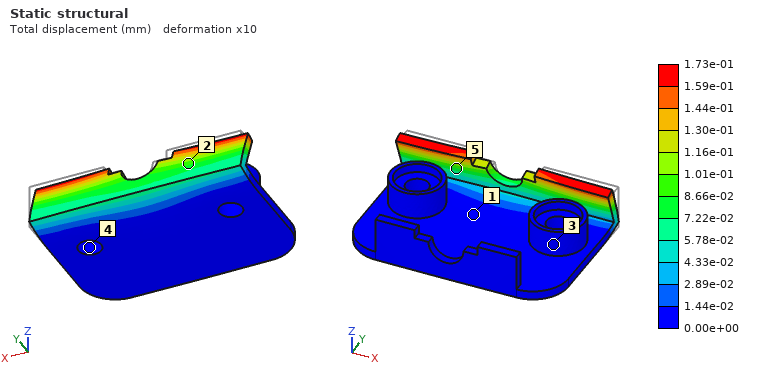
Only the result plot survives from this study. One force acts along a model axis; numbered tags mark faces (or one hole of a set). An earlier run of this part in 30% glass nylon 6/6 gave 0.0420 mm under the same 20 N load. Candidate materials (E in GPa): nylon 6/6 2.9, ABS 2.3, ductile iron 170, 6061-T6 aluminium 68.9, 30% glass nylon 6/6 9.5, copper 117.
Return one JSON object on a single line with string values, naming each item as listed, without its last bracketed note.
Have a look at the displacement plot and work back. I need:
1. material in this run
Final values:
{"material in this run": "ABS"}
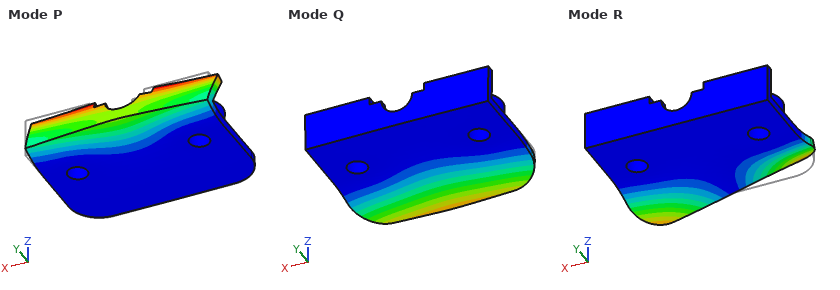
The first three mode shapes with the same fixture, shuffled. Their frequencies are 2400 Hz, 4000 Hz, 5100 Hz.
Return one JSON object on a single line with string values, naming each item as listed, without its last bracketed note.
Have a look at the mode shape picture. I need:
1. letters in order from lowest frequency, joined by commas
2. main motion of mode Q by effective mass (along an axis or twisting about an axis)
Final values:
{"letters in order from lowest frequency, joined by commas": "Q, R, P", "main motion of mode Q by effective mass": "along Z"}
